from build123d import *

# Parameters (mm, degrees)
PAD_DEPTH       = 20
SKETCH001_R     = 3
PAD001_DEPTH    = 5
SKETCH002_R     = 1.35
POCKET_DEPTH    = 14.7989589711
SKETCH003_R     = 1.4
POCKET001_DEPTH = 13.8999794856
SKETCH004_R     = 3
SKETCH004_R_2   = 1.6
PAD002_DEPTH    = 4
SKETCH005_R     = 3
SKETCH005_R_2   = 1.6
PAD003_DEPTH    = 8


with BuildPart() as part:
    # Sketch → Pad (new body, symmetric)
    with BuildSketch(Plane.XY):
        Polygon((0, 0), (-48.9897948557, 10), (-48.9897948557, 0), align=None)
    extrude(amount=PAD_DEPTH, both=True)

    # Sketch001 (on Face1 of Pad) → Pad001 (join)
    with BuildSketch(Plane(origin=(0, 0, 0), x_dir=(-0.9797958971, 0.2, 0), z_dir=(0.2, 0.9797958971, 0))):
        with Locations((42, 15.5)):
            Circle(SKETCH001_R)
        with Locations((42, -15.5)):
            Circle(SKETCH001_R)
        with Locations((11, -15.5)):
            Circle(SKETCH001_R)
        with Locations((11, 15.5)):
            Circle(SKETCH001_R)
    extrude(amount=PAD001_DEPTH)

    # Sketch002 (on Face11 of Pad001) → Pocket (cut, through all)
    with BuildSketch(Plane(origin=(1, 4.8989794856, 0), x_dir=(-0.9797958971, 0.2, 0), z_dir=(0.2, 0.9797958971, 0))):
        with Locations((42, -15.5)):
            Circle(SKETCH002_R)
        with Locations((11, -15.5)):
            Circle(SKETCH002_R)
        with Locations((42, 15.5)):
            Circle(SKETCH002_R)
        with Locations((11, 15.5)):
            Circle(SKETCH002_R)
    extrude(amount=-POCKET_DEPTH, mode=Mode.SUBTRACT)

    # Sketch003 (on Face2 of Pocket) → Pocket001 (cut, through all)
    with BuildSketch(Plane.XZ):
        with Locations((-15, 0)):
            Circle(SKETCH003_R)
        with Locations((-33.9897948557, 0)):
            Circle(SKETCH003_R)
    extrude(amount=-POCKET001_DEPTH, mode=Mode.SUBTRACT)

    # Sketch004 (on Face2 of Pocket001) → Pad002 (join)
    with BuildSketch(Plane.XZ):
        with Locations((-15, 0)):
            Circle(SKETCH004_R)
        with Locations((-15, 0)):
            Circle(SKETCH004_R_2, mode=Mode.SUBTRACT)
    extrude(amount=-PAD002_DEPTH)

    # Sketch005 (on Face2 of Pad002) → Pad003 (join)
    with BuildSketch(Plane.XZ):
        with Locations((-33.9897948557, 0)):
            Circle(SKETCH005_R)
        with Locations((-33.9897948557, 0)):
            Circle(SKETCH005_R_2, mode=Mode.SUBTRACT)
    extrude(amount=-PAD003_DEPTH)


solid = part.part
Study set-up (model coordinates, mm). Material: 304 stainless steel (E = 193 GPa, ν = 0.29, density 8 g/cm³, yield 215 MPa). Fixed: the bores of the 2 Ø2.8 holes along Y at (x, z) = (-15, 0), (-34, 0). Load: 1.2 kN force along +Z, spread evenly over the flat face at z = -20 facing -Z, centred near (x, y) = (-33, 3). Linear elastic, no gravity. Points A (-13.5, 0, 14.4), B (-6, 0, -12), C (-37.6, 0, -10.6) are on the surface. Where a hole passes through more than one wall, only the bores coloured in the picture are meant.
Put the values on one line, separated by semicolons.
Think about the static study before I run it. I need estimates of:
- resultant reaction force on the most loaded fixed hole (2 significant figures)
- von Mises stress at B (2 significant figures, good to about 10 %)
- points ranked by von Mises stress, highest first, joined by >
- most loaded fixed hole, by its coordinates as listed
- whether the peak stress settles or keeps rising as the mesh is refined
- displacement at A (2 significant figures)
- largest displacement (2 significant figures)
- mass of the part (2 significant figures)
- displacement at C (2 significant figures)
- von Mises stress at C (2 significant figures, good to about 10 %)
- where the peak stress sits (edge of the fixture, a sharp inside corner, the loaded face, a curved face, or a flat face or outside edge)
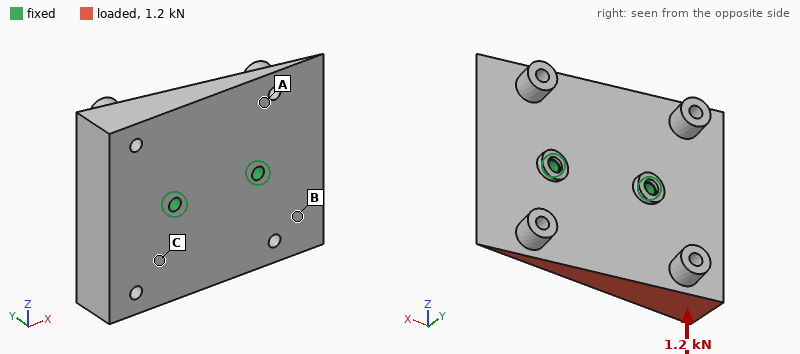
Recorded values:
1.1 kN; 4.9 MPa; C > B > A; (-34, 0); keeps rising; 0.32 µm; 1.6 µm; 81 g; 0.79 µm; 7.1 MPa; edge of the fixture
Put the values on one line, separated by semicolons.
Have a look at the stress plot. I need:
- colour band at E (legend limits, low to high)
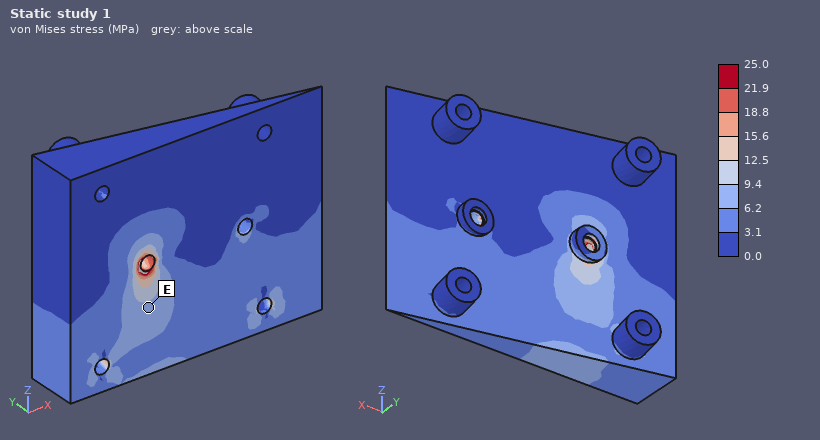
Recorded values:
6.2 to 9.4 MPa
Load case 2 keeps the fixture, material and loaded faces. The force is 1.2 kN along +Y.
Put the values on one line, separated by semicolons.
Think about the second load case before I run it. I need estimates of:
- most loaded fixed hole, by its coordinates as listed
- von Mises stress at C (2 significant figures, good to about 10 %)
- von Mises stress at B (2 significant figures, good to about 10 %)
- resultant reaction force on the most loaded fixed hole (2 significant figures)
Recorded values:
(-34, 0); 42 MPa; 25 MPa; 1.1 kN
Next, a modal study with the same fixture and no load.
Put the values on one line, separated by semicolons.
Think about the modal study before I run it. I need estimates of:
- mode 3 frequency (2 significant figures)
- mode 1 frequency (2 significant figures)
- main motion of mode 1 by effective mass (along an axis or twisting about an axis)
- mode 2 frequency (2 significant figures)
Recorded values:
9300 Hz; 7000 Hz; twisting about X; 8600 Hz
